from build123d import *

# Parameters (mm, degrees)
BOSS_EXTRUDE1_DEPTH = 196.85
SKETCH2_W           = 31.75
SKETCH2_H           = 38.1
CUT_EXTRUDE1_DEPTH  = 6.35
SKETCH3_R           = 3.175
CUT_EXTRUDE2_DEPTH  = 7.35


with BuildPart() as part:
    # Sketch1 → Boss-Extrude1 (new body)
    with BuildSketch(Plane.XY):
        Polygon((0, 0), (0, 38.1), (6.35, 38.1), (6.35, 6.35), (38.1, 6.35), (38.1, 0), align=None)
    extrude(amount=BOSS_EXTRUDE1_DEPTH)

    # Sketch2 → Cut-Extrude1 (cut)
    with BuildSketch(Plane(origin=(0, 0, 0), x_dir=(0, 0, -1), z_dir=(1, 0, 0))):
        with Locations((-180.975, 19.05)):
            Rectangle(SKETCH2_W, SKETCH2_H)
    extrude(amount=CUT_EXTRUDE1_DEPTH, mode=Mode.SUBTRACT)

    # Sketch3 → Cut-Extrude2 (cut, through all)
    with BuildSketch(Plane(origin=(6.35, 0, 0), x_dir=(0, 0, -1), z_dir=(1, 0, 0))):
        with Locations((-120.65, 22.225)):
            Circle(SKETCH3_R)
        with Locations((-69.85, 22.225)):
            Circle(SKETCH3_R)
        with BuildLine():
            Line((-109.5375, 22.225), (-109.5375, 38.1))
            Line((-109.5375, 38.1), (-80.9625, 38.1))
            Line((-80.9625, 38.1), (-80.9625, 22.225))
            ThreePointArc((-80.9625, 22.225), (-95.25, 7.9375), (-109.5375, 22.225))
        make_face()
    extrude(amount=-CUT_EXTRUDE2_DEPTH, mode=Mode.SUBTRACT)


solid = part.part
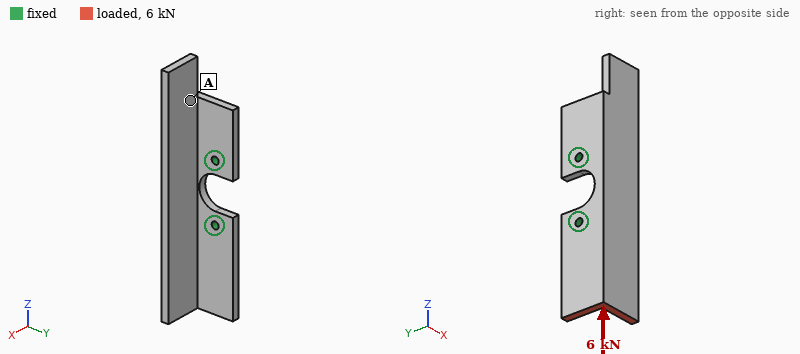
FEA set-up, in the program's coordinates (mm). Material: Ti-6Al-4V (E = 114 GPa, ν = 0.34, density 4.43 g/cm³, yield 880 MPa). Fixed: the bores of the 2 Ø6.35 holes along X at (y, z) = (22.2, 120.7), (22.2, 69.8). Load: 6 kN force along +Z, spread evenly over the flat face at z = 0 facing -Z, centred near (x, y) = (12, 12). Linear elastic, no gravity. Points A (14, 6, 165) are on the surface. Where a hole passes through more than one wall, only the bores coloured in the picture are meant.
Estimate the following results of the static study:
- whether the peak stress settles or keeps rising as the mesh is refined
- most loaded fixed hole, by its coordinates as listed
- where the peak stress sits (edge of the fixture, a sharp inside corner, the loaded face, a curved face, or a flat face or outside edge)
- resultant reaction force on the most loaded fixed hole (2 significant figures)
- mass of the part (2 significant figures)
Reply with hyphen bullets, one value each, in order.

- keeps rising
- (22.2, 69.8)
- edge of the fixture
- 4.5 kN
- 330 g
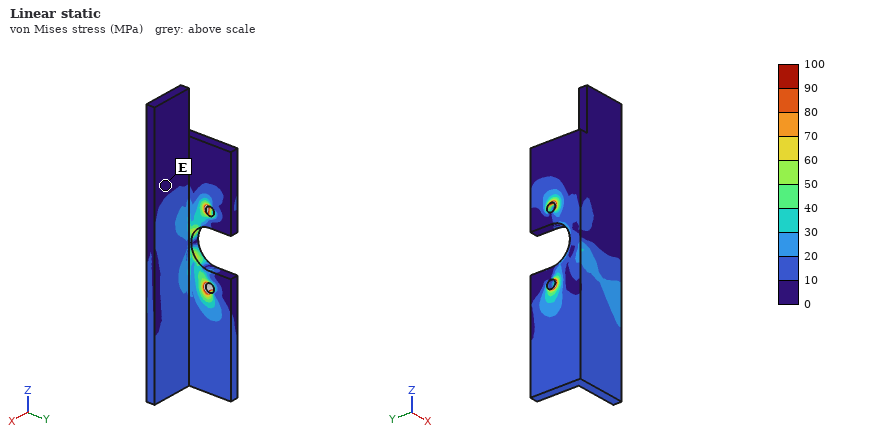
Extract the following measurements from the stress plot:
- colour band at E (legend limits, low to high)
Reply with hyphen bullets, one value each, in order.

- 0 to 10 MPa
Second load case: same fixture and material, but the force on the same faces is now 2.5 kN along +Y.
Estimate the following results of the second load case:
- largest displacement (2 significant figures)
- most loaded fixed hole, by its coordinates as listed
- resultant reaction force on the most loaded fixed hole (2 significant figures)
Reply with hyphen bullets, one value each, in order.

- 0.52 mm
- (22.2, 69.8)
- 5.3 kN
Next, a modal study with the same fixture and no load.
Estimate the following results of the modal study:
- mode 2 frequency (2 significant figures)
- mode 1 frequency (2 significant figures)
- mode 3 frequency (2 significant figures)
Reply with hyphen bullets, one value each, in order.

- 1500 Hz
- 1300 Hz
- 1900 Hz
